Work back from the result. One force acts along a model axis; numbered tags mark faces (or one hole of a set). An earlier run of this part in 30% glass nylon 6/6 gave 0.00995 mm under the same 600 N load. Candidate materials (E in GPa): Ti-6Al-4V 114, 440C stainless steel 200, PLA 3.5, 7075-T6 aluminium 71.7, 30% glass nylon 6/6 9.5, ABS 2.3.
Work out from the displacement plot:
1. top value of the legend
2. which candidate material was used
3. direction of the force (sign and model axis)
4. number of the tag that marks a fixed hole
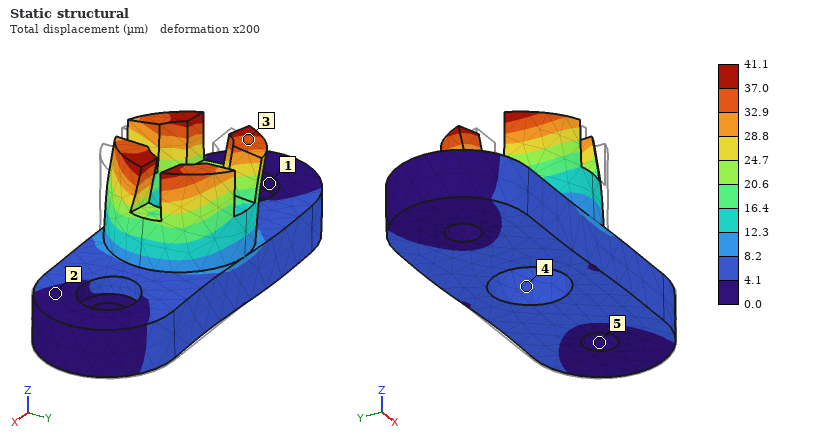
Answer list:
41.1 µm
ABS
-X
5
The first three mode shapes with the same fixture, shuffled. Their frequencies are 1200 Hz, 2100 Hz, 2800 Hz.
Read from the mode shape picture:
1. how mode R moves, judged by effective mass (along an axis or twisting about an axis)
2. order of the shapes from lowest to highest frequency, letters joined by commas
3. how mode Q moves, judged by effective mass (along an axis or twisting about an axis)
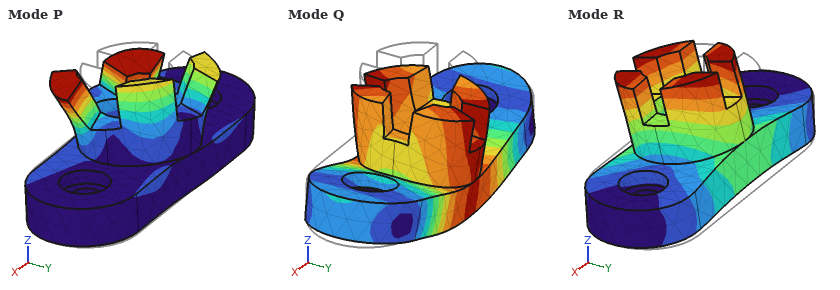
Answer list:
along Y
R, Q, P
along Z
